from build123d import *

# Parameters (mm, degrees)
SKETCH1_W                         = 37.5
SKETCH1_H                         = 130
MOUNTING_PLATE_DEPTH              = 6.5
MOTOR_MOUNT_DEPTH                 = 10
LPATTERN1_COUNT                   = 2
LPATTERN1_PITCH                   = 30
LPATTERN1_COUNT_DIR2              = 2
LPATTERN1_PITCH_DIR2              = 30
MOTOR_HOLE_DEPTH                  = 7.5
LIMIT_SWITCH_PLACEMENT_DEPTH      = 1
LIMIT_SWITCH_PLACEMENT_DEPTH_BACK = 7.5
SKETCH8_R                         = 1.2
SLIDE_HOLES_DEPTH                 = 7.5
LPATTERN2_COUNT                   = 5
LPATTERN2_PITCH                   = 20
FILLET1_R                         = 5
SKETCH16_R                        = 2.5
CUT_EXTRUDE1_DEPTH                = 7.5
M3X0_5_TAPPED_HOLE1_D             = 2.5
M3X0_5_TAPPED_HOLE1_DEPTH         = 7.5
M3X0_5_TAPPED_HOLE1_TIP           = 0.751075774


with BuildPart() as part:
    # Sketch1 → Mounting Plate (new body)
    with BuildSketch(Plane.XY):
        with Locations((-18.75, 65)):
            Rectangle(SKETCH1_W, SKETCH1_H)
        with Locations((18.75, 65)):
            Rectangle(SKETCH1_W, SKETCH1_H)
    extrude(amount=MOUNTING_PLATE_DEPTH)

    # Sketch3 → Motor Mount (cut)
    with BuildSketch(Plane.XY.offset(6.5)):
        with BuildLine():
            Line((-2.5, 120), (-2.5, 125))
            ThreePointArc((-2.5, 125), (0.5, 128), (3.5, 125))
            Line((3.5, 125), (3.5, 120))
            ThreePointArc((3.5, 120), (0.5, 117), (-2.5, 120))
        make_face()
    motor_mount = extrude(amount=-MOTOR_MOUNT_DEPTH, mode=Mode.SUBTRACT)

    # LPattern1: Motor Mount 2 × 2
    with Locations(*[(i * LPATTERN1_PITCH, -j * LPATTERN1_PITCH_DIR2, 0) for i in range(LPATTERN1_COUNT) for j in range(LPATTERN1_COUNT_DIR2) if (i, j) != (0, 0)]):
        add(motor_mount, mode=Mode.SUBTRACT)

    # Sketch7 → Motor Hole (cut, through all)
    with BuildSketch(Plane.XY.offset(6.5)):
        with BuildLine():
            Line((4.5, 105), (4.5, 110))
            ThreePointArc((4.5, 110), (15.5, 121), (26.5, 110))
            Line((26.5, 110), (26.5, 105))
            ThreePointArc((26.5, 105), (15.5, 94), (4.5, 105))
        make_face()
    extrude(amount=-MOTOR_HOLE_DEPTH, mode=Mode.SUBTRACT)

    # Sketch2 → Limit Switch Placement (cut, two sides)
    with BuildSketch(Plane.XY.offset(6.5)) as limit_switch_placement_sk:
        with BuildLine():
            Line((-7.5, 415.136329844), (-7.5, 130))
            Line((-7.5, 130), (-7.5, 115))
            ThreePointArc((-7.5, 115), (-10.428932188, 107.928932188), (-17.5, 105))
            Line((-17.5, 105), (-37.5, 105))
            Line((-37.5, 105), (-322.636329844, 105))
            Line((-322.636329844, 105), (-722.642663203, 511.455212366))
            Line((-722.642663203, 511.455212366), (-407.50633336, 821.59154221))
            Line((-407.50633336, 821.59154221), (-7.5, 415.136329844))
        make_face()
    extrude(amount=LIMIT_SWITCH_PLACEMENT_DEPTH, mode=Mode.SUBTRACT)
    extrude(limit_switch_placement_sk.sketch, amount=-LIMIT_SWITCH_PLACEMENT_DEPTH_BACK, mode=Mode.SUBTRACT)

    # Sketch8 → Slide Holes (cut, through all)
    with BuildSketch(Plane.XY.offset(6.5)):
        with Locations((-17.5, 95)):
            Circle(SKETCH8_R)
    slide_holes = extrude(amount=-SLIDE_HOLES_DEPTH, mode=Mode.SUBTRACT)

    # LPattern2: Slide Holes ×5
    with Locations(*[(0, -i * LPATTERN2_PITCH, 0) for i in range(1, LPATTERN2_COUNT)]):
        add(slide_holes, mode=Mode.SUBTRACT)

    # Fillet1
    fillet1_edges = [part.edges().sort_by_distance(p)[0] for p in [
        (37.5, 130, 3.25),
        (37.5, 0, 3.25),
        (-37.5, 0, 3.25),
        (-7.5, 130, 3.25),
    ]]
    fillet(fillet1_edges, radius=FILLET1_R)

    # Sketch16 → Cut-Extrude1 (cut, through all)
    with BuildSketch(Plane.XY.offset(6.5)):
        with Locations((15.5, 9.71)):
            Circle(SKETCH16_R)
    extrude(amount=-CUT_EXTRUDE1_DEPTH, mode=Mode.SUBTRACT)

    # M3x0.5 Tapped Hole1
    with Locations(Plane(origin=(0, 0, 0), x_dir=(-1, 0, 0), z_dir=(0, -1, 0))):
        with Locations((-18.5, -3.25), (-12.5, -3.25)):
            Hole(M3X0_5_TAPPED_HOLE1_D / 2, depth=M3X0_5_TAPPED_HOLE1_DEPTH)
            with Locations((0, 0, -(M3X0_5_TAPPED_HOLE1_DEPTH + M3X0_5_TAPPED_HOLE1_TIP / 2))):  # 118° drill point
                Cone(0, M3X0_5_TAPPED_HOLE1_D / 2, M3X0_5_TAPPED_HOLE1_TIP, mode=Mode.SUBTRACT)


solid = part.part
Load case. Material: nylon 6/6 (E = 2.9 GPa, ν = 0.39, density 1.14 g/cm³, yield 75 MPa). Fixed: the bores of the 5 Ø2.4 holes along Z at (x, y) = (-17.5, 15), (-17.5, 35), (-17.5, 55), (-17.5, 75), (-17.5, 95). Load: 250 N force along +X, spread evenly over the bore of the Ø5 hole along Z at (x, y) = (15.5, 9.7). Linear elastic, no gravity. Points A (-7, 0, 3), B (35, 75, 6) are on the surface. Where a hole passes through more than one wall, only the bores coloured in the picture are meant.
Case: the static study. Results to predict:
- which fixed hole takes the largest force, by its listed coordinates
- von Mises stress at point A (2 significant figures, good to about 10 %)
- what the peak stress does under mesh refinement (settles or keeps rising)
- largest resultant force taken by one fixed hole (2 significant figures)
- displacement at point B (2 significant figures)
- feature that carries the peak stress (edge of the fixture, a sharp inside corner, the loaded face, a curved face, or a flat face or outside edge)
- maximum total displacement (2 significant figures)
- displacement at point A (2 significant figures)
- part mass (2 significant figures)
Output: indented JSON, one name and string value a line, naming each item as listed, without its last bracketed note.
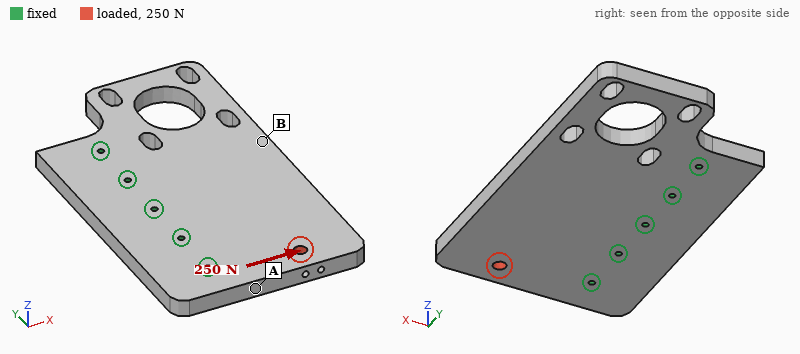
{
  "which fixed hole takes the largest force, by its listed coordinates": "(-17.5, 15)",
  "von Mises stress at point A": "0.94 MPa",
  "what the peak stress does under mesh refinement": "keeps rising",
  "largest resultant force taken by one fixed hole": "210 N",
  "displacement at point B": "10 µm",
  "feature that carries the peak stress": "edge of the fixture",
  "maximum total displacement": "33 µm",
  "displacement at point A": "16 µm",
  "part mass": "61 g"
}
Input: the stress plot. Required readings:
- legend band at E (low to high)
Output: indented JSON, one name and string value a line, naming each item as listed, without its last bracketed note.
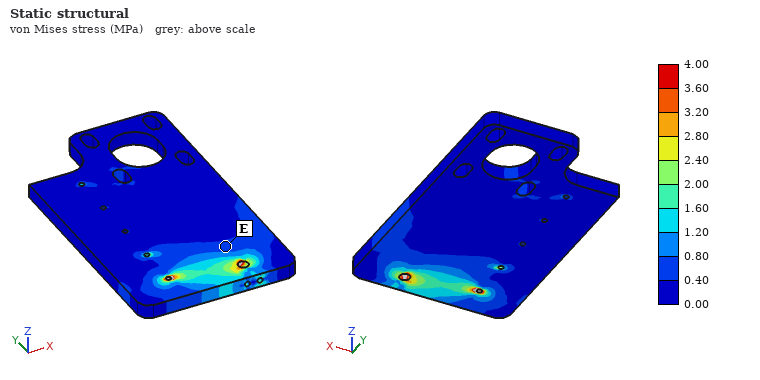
{
  "legend band at E": "0.40 to 0.80 MPa"
}
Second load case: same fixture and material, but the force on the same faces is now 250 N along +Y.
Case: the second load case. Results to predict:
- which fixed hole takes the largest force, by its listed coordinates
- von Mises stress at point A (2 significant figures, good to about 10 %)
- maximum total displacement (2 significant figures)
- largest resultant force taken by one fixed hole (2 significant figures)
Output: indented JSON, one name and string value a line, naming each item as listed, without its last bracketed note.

{
  "which fixed hole takes the largest force, by its listed coordinates": "(-17.5, 15)",
  "von Mises stress at point A": "0.66 MPa",
  "maximum total displacement": "38 µm",
  "largest resultant force taken by one fixed hole": "130 N"
}
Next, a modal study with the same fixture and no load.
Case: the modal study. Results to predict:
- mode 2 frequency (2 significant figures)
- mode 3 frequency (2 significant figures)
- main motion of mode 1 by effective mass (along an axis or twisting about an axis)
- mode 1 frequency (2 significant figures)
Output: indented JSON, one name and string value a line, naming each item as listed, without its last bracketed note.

{
  "mode 2 frequency": "620 Hz",
  "mode 3 frequency": "1000 Hz",
  "main motion of mode 1 by effective mass": "along Z",
  "mode 1 frequency": "470 Hz"
}
